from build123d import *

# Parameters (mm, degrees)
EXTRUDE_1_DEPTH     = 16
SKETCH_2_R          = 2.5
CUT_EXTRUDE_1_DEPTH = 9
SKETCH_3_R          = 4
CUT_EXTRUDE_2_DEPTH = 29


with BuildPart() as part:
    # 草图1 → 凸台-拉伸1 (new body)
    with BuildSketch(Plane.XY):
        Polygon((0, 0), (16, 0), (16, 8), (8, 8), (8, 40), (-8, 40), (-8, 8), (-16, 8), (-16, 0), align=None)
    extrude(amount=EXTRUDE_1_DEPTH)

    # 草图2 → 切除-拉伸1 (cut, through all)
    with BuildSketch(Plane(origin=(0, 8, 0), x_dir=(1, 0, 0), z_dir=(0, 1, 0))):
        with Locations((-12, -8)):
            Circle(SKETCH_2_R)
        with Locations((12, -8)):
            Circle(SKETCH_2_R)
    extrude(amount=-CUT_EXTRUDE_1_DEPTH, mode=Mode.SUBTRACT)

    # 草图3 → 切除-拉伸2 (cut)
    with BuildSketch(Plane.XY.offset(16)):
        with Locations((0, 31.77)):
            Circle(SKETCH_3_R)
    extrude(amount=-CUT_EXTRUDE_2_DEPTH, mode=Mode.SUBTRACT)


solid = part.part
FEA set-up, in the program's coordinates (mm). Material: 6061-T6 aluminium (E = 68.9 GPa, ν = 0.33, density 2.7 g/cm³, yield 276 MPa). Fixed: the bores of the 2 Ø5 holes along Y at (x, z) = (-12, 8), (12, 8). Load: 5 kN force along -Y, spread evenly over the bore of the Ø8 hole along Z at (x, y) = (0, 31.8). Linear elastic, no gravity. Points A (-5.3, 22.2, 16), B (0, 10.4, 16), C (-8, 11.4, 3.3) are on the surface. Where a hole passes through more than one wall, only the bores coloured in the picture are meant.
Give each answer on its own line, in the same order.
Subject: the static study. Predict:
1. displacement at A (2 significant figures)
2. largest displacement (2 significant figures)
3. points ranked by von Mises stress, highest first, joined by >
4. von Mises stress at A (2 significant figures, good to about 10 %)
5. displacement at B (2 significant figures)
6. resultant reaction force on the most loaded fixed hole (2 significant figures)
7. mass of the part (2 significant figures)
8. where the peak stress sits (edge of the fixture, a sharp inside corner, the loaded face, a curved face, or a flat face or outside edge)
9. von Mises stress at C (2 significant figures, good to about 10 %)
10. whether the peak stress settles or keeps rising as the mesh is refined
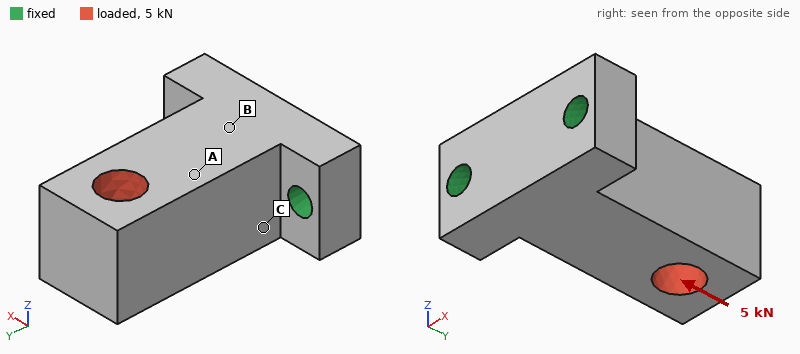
10 µm
18 µm
C > A > B
21 MPa
7.7 µm
2.6 kN
30 g
edge of the fixture
28 MPa
keeps rising
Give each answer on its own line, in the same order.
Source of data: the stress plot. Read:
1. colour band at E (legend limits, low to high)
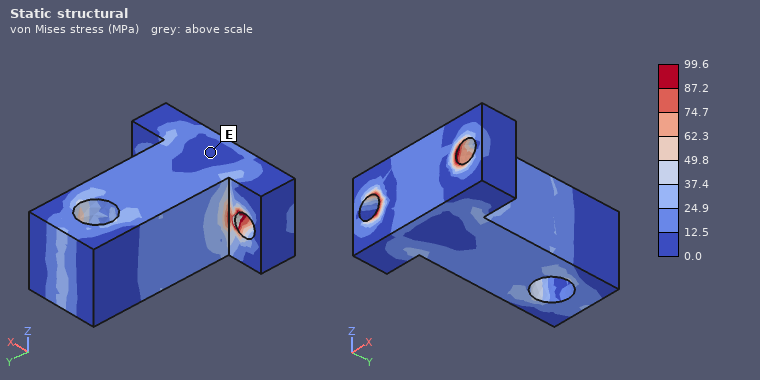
0.0 to 12.5 MPa
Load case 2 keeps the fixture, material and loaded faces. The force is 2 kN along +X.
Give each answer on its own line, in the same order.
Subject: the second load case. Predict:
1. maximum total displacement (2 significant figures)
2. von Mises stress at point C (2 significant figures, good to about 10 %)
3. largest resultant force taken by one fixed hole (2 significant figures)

79 µm
63 MPa
2.9 kN
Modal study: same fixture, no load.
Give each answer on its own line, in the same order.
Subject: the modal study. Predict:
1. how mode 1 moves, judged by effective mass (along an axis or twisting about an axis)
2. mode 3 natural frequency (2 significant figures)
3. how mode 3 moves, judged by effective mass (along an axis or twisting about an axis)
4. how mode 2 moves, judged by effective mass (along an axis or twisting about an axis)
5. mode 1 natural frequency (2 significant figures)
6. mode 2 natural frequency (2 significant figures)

along Z
20 kHz
twisting about Y
along X
5900 Hz
9000 Hz
